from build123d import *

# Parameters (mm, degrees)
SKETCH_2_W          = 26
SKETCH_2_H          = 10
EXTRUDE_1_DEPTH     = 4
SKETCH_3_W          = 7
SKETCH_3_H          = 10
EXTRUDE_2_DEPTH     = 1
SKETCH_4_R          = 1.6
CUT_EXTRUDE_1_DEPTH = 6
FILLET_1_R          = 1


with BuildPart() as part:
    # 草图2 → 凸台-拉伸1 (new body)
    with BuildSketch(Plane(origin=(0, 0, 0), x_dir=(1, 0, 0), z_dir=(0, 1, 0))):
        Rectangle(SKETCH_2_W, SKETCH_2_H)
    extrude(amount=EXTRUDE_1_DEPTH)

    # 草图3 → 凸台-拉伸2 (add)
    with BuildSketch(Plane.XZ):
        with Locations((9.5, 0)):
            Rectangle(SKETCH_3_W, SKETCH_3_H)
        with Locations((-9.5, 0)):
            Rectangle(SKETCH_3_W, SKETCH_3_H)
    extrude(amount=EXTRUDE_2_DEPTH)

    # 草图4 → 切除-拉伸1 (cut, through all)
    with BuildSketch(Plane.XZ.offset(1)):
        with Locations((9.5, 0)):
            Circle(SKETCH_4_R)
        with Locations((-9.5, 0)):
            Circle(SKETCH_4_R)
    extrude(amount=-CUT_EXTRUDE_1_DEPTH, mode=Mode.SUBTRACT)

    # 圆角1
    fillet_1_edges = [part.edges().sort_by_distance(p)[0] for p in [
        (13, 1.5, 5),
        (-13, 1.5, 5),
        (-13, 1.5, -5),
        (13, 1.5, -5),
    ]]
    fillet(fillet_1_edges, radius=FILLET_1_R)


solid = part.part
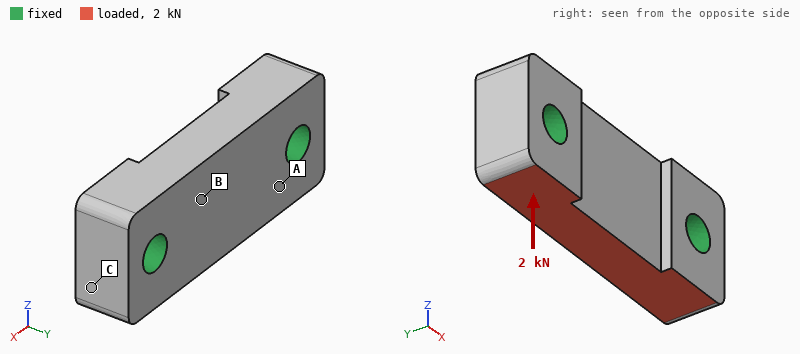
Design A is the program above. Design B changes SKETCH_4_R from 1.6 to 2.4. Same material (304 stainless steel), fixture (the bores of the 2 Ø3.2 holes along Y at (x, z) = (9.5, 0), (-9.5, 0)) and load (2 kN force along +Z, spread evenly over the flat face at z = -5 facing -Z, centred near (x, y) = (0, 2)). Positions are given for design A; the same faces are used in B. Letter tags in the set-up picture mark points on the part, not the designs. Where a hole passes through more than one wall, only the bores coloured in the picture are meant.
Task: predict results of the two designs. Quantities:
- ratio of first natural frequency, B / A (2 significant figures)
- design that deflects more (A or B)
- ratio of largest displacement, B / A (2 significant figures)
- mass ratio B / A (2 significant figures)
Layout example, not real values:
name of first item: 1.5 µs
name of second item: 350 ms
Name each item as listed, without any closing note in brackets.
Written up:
ratio of first natural frequency, B / A: 1.2
design that deflects more: A
ratio of largest displacement, B / A: 0.75
mass ratio B / A: 0.91
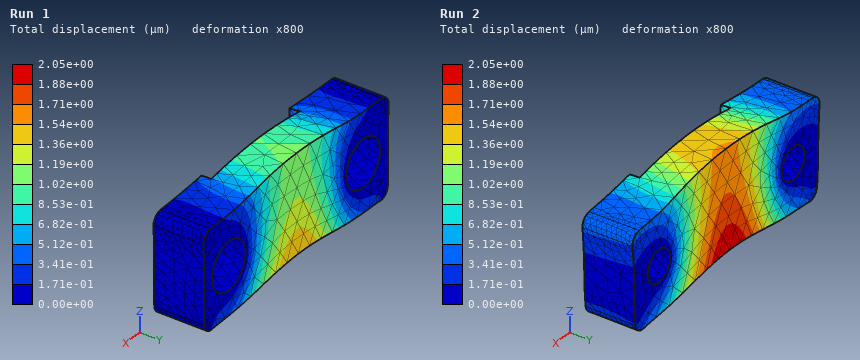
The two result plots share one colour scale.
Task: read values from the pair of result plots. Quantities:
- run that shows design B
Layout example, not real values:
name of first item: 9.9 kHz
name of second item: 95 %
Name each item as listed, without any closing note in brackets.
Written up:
run that shows design B: Run 1
